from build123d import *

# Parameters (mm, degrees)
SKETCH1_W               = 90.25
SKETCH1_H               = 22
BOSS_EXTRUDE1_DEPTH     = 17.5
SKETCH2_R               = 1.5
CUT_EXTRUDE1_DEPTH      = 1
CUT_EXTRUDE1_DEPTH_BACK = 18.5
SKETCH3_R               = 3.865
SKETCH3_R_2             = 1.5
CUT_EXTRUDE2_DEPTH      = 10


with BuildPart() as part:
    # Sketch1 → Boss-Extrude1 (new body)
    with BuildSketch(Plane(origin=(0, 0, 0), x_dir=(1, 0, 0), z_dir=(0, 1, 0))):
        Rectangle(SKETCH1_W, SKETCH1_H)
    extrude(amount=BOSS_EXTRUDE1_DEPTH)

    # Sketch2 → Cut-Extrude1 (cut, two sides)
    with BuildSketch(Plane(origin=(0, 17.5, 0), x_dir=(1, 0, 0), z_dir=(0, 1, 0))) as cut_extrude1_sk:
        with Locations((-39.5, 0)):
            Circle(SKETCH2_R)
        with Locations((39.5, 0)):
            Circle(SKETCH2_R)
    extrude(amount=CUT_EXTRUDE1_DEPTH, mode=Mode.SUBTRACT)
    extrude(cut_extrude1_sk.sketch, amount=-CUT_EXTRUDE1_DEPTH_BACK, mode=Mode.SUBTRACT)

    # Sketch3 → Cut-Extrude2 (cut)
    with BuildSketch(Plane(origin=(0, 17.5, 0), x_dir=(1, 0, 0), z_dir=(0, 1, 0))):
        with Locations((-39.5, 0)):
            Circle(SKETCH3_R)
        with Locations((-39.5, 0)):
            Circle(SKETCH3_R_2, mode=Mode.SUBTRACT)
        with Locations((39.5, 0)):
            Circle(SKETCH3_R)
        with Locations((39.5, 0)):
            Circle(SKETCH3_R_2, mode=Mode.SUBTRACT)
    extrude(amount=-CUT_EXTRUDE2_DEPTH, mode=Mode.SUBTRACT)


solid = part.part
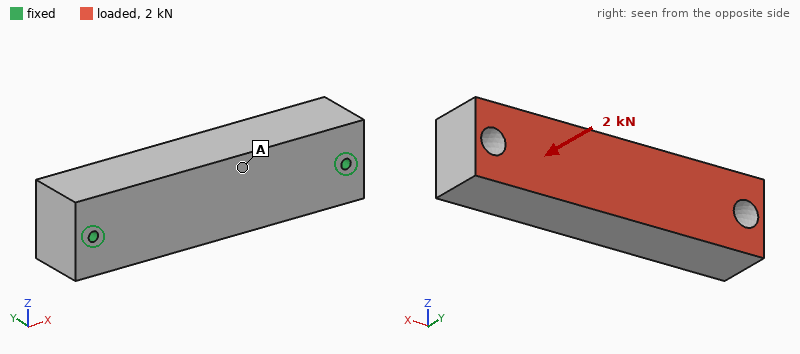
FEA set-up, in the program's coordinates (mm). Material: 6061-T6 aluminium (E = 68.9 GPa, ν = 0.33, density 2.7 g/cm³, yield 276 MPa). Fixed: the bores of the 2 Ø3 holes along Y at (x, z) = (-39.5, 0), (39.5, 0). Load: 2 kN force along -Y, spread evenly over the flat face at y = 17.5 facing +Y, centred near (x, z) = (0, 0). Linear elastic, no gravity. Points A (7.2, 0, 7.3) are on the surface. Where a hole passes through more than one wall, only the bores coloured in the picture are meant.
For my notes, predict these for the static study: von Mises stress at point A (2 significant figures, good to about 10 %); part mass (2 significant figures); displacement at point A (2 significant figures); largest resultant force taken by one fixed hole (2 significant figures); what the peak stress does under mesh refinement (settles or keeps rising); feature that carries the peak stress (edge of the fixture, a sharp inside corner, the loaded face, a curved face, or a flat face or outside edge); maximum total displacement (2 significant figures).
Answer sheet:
7.5 MPa
91 g
12 µm
1.2 kN
keeps rising
edge of the fixture
13 µm
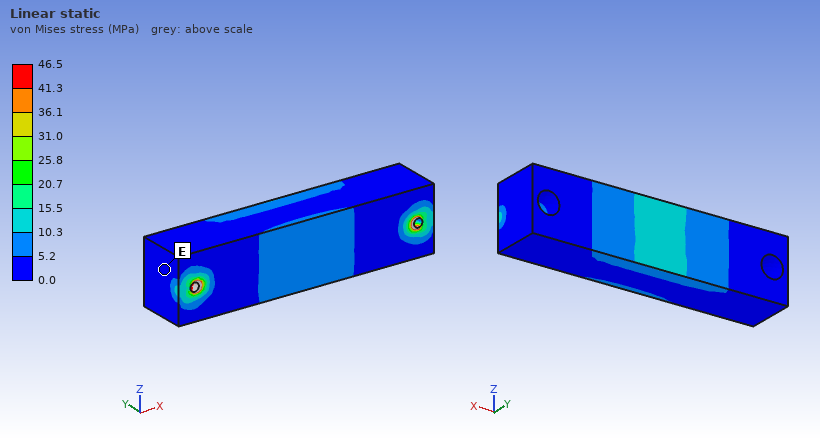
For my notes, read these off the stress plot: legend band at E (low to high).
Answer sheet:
0.0 to 5.2 MPa
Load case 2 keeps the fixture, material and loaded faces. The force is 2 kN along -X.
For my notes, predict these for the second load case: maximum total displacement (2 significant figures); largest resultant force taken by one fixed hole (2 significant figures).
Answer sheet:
3.3 µm
1.1 kN
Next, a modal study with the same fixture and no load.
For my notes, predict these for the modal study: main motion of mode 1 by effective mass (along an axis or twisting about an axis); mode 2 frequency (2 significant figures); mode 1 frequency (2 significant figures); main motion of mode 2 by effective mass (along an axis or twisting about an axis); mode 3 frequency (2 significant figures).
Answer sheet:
along Z
7400 Hz
6300 Hz
along Y
9600 Hz
